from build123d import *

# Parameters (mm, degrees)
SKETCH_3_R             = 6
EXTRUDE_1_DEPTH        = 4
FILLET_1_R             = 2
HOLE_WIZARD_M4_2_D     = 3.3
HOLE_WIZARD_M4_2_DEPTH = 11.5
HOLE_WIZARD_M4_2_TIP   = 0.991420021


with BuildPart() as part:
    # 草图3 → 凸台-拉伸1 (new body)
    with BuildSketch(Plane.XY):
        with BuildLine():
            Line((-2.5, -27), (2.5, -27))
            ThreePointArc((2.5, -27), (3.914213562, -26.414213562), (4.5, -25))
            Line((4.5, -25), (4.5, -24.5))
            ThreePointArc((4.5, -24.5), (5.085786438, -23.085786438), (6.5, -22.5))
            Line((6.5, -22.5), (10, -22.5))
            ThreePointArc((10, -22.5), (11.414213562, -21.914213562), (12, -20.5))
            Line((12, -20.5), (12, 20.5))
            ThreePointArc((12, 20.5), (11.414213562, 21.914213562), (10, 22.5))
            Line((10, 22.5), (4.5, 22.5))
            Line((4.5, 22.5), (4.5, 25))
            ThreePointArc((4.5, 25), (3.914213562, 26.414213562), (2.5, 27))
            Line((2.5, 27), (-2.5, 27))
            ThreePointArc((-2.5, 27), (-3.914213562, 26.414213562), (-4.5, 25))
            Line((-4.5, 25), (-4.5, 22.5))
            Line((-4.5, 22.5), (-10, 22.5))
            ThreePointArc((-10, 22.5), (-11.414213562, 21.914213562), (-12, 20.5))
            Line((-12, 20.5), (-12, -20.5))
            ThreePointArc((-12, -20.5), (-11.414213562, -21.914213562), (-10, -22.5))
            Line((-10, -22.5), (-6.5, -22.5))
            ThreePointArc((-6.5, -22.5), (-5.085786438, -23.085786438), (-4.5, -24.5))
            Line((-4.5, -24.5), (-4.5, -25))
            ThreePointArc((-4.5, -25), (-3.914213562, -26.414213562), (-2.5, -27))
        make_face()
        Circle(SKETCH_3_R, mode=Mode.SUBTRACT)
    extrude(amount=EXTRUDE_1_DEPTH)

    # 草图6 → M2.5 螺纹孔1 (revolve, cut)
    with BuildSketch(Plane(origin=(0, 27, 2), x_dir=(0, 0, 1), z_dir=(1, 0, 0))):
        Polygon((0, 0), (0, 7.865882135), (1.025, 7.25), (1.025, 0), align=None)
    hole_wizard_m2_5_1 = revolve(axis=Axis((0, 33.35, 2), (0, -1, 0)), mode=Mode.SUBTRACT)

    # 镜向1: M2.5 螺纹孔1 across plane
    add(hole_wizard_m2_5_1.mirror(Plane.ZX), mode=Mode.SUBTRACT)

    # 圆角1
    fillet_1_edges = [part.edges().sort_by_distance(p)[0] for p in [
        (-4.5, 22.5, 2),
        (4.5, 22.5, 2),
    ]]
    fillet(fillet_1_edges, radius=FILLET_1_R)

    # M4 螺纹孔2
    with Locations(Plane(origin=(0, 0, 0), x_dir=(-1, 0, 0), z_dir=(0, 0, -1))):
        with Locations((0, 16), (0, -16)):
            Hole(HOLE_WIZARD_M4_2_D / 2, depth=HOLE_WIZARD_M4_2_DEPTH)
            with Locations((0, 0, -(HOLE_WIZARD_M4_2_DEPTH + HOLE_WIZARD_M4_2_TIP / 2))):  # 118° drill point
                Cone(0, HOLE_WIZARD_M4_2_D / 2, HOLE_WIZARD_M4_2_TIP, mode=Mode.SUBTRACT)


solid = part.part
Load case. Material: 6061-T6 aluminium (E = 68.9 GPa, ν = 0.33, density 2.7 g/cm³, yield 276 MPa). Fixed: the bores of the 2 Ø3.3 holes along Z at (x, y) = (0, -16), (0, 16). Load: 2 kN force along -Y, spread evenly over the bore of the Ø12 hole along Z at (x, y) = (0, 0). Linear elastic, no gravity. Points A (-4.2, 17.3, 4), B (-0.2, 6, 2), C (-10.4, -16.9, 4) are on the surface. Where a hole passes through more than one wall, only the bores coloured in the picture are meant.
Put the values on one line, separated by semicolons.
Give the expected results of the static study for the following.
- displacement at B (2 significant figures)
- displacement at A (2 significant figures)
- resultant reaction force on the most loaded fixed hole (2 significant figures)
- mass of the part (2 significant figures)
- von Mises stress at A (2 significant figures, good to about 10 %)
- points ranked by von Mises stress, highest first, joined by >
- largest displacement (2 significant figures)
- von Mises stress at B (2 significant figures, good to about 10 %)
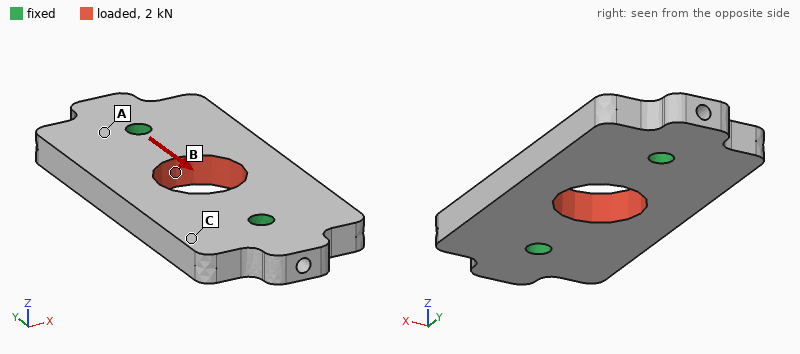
2.7 µm; 1.1 µm; 1.0 kN; 11 g; 9.1 MPa; B > A > C; 4.4 µm; 20 MPa
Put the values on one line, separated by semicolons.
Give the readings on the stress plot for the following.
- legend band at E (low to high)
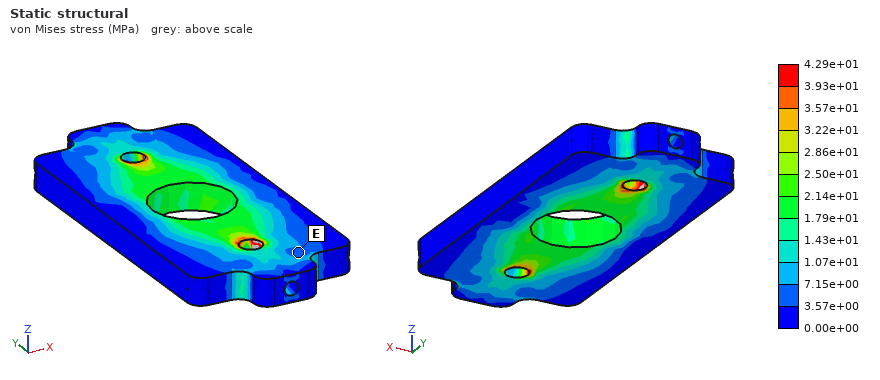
3.57e+00 to 7.15e+00 MPa
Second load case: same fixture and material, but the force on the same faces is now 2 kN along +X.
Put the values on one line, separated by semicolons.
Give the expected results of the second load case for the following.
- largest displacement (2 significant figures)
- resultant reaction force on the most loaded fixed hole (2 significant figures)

11 µm; 1.0 kN
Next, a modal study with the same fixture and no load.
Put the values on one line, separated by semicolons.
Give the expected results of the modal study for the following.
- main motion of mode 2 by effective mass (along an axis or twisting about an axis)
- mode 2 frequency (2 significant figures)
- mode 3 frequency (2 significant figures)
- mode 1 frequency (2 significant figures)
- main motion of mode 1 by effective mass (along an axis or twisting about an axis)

along Z; 15 kHz; 22 kHz; 14 kHz; twisting about Y
